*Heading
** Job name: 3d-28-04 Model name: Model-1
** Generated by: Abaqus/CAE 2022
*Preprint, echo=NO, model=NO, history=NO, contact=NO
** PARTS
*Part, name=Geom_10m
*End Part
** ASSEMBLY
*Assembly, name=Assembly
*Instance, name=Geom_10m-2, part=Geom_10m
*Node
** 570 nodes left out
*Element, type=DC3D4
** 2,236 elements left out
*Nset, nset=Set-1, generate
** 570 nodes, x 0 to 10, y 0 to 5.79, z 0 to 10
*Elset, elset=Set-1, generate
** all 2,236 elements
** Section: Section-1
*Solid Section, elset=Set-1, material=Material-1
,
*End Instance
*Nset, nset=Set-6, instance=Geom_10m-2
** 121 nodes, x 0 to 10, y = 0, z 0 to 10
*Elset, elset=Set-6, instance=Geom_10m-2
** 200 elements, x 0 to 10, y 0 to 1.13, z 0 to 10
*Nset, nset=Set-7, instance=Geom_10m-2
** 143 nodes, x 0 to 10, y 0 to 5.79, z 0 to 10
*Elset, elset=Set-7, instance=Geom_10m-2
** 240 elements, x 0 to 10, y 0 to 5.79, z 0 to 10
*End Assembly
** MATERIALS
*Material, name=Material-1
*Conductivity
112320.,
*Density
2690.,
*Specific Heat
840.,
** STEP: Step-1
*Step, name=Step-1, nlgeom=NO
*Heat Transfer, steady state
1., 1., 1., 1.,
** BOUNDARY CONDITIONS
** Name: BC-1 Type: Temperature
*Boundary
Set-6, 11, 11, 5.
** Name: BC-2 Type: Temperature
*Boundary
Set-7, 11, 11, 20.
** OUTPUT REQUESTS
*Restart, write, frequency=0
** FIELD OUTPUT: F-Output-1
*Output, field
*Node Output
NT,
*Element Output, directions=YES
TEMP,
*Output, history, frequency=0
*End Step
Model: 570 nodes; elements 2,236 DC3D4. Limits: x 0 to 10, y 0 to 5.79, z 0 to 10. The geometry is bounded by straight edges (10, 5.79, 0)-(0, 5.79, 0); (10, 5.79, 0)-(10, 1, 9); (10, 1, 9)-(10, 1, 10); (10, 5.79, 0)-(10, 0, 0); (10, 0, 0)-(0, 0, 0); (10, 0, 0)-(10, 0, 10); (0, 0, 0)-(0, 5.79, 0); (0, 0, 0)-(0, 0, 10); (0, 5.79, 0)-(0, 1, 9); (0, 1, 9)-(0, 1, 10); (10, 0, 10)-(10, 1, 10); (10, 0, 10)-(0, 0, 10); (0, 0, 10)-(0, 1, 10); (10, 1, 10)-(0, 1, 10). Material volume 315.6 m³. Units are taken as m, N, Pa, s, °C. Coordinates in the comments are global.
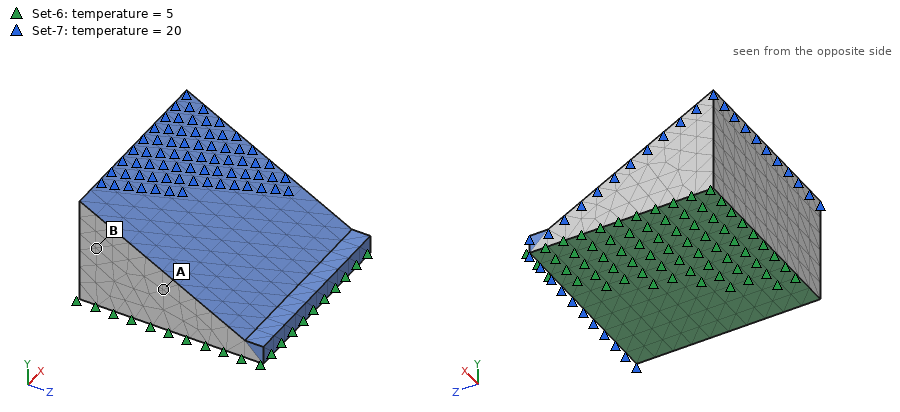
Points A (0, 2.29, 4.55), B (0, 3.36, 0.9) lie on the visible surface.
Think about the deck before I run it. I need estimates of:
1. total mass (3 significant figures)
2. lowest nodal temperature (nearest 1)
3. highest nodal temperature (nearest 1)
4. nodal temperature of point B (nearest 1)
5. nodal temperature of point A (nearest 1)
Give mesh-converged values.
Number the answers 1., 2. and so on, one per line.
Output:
1. 8.49e+05 kg
2. 5 °C
3. 20 °C
4. 16 °C
5. 16 °C
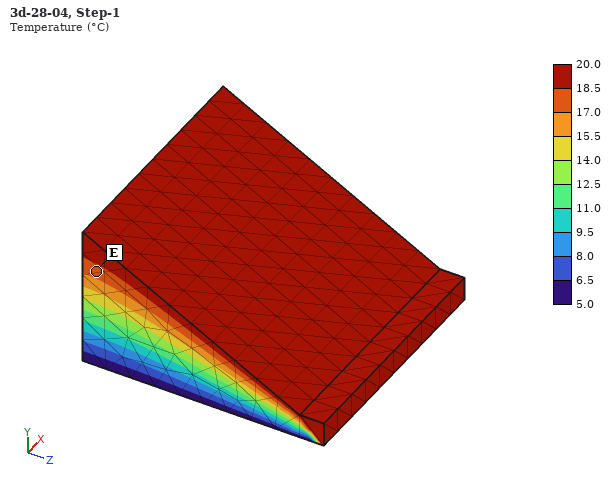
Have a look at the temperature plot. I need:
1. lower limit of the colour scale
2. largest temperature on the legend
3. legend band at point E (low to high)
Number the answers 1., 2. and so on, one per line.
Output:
1. 5.0 °C
2. 20.0 °C
3. 17.0 to 18.5 °C
